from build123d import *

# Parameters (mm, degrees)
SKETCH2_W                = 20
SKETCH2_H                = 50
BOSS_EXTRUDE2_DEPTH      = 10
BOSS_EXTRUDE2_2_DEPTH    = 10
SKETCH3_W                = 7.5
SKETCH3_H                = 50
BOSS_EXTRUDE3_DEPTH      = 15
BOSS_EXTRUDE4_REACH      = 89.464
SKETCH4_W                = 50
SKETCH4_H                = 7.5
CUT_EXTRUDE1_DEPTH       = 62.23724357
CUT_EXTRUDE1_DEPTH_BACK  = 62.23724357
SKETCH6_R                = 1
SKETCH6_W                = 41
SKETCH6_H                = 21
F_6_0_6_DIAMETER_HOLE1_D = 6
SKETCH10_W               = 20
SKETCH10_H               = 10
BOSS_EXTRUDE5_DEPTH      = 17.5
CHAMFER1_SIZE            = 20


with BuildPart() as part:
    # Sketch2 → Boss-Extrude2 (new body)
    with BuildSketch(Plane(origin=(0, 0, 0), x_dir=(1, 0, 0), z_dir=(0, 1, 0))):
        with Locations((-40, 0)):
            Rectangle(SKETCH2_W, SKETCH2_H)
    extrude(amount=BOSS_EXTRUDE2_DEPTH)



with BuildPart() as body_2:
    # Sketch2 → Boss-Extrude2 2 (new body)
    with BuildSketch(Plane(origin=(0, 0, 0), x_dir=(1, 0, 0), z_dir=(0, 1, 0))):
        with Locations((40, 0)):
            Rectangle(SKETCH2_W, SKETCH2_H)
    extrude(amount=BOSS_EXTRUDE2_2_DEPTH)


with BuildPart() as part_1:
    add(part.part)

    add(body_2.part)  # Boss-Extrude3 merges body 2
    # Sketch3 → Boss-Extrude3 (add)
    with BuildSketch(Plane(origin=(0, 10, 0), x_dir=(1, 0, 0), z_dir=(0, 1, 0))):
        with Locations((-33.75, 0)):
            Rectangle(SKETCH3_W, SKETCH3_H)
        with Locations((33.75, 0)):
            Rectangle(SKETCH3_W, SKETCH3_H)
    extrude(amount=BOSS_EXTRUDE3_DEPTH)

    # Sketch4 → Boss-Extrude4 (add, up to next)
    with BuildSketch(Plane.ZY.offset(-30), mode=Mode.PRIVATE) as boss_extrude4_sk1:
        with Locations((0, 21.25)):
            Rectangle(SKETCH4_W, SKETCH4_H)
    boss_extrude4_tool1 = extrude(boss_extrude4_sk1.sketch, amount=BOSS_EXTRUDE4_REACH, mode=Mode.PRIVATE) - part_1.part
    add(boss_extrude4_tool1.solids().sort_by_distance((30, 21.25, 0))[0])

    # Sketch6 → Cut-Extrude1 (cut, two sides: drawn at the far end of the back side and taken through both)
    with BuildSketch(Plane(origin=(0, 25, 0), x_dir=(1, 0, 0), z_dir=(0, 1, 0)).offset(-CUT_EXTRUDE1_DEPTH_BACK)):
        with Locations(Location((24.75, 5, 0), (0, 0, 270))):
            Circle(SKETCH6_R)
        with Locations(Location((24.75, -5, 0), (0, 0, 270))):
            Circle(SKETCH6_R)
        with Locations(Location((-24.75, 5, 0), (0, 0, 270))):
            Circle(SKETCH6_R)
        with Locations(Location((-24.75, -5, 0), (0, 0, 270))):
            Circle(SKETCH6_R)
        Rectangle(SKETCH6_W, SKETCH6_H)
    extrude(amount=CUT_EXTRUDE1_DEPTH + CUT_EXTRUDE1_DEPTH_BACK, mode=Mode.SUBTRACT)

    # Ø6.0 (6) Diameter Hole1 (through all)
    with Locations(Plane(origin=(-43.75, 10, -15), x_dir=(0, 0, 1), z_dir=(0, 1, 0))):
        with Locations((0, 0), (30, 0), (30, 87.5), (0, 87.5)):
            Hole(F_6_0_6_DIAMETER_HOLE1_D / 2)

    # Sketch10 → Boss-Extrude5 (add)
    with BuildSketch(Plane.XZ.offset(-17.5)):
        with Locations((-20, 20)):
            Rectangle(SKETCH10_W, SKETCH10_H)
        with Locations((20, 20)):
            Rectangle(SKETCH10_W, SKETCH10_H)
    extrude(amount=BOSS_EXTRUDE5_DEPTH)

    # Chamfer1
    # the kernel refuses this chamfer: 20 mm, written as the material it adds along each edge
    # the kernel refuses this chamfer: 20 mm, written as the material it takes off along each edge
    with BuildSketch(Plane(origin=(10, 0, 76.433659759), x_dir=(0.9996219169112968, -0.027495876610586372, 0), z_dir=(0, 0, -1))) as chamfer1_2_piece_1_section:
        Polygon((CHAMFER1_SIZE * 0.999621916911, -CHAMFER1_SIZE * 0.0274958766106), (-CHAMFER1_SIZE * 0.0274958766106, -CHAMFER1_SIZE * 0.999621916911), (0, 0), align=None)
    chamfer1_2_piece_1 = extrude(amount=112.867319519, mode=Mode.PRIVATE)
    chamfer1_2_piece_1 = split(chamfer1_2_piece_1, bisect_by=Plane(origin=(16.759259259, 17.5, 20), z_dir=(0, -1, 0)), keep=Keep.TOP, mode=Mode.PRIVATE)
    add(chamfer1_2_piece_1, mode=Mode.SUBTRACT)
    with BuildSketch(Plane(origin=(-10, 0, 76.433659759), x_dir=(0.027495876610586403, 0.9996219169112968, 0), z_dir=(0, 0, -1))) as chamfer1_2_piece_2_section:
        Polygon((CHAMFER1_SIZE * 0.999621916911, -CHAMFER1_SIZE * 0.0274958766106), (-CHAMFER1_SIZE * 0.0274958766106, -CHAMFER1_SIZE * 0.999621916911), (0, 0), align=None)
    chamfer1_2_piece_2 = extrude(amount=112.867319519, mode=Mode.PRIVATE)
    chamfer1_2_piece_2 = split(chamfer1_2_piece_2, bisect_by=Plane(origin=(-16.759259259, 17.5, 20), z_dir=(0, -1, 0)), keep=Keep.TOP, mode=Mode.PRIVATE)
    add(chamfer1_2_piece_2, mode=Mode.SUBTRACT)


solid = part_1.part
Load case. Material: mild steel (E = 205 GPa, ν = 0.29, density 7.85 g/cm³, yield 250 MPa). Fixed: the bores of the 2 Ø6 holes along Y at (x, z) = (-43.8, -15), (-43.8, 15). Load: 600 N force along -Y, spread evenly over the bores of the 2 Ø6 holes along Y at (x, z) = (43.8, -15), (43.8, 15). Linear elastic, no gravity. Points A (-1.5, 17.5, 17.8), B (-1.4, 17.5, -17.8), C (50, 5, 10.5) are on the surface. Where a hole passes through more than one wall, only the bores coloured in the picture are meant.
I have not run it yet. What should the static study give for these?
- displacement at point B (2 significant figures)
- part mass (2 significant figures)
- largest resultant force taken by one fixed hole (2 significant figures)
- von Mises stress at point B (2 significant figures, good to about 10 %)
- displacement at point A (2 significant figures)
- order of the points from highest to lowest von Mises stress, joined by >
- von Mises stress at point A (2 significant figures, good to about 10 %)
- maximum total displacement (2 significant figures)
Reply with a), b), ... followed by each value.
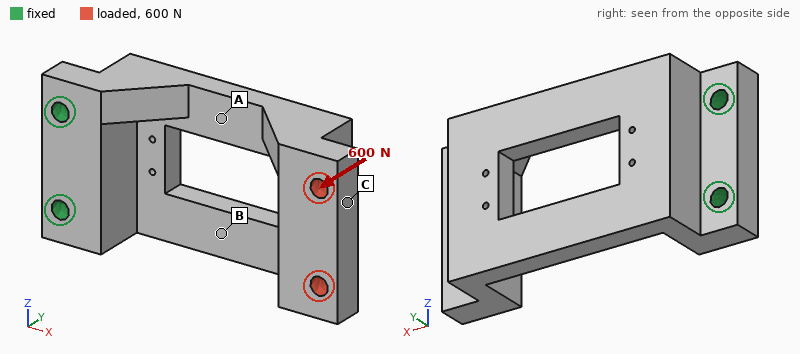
a) 0.11 mm
b) 390 g
c) 380 N
d) 76 MPa
e) 0.079 mm
f) A > B > C
g) 120 MPa
h) 0.48 mm
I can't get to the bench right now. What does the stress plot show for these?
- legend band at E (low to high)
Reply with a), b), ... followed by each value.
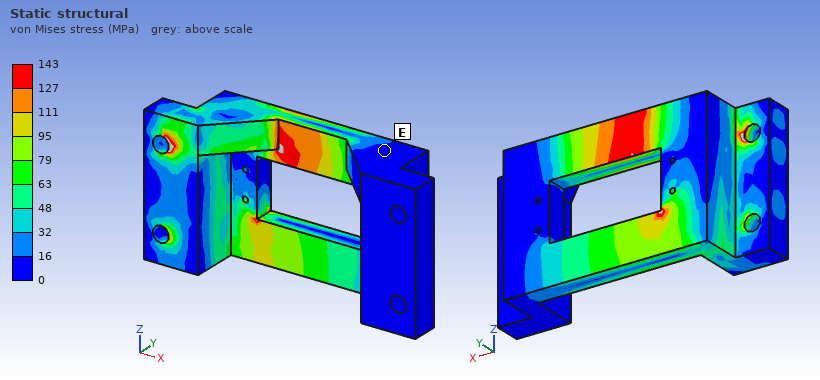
a) 0 to 16 MPa
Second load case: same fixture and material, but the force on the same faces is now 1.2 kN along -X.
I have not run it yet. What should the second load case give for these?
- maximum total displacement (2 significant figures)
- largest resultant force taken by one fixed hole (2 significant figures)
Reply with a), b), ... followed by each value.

a) 0.25 mm
b) 600 N
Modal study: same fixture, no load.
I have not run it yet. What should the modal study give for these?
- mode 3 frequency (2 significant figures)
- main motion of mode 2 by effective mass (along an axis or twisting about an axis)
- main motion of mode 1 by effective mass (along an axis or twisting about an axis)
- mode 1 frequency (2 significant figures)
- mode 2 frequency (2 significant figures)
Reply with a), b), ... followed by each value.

a) 2500 Hz
b) along Z
c) along Y
d) 560 Hz
e) 1200 Hz
